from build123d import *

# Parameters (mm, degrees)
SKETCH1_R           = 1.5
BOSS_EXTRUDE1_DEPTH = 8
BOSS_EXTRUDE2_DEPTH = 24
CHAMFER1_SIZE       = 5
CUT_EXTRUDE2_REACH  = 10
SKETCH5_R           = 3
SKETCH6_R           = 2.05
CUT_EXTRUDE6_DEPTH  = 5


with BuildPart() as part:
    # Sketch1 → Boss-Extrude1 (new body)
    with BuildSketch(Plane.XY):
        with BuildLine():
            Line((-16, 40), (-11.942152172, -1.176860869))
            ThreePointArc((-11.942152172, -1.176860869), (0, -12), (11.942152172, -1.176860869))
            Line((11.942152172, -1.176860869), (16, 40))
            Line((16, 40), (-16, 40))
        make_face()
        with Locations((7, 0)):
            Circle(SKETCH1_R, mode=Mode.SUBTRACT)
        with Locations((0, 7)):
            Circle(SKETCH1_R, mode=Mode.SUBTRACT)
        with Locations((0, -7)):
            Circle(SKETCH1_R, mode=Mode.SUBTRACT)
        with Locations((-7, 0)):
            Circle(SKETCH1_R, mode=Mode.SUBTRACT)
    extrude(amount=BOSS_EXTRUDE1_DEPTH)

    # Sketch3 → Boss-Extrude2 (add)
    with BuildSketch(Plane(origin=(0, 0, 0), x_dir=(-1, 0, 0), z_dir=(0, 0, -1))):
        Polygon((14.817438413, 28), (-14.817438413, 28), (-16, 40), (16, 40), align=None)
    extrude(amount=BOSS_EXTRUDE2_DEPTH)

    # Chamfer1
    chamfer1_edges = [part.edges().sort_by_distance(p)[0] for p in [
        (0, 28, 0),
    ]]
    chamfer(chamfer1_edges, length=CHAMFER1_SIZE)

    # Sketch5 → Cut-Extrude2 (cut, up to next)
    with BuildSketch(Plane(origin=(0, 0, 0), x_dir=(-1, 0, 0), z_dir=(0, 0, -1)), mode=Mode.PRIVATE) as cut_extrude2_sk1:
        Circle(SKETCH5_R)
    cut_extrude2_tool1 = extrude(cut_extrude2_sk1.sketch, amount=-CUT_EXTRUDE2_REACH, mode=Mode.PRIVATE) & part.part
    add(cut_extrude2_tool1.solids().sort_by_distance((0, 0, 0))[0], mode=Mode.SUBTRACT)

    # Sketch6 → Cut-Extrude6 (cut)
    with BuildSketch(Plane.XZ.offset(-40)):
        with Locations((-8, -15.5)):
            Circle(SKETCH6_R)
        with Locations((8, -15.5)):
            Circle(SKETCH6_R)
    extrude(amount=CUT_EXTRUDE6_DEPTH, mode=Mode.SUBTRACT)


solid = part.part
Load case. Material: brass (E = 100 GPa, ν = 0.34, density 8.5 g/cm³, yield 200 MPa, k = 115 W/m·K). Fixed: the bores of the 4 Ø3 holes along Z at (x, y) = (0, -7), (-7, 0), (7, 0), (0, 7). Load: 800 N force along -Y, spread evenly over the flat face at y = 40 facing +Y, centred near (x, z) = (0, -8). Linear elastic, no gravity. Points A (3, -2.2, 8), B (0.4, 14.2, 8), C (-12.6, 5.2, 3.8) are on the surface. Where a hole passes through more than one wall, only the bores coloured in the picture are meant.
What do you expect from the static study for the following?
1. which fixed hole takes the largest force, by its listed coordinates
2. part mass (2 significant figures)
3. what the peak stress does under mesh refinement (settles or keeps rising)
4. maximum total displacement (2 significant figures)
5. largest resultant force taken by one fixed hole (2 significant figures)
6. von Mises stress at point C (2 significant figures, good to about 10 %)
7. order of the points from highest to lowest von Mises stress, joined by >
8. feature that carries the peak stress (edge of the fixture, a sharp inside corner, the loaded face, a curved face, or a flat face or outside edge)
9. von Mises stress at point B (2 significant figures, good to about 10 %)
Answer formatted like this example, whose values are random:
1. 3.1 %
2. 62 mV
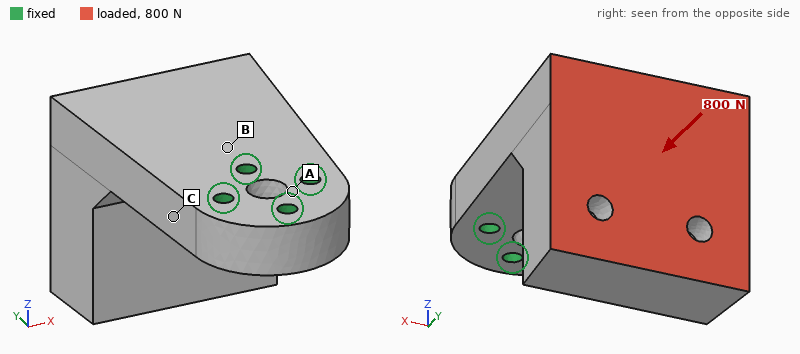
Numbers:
1. (0, 7)
2. 170 g
3. keeps rising
4. 67 µm
5. 590 N
6. 13 MPa
7. B > C > A
8. edge of the fixture
9. 29 MPa
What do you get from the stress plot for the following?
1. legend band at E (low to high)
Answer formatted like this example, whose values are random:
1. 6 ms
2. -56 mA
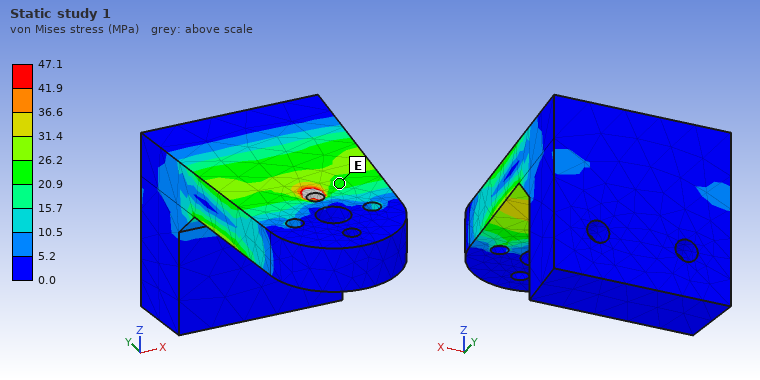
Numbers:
1. 20.9 to 26.2 MPa
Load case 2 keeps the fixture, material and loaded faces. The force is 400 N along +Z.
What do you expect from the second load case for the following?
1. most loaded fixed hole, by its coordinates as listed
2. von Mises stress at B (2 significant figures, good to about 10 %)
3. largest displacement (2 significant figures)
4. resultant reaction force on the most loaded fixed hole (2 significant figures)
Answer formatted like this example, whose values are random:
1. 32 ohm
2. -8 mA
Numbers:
1. (0, 7)
2. 37 MPa
3. 70 µm
4. 860 N
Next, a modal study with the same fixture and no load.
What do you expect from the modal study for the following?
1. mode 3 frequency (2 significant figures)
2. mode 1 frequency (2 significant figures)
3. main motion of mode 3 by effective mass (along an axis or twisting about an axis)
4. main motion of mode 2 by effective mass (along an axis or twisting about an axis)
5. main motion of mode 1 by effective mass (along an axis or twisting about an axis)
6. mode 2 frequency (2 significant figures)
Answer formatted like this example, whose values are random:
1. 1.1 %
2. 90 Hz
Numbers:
1. 5000 Hz
2. 1500 Hz
3. along X
4. along X
5. along Z
6. 2300 Hz
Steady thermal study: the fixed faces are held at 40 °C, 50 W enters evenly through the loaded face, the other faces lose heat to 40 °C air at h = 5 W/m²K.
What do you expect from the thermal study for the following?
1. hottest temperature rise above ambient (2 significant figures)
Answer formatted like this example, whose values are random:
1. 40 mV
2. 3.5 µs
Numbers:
1. 62 K
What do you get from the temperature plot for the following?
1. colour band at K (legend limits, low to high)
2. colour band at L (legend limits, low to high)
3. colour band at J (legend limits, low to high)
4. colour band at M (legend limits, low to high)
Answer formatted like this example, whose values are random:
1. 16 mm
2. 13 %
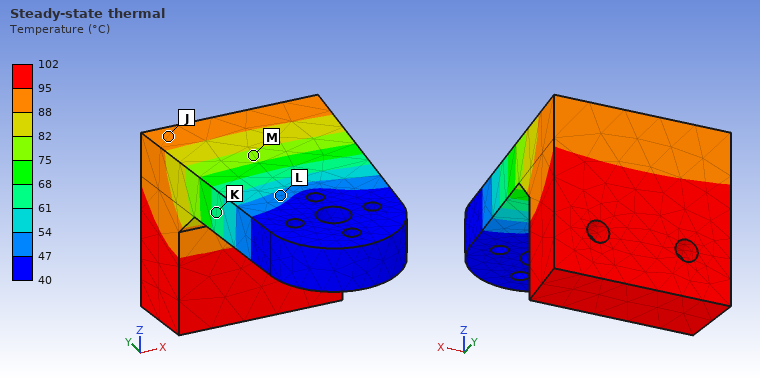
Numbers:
1. 61 to 68 °C
2. 47 to 54 °C
3. 88 to 95 °C
4. 75 to 82 °C
